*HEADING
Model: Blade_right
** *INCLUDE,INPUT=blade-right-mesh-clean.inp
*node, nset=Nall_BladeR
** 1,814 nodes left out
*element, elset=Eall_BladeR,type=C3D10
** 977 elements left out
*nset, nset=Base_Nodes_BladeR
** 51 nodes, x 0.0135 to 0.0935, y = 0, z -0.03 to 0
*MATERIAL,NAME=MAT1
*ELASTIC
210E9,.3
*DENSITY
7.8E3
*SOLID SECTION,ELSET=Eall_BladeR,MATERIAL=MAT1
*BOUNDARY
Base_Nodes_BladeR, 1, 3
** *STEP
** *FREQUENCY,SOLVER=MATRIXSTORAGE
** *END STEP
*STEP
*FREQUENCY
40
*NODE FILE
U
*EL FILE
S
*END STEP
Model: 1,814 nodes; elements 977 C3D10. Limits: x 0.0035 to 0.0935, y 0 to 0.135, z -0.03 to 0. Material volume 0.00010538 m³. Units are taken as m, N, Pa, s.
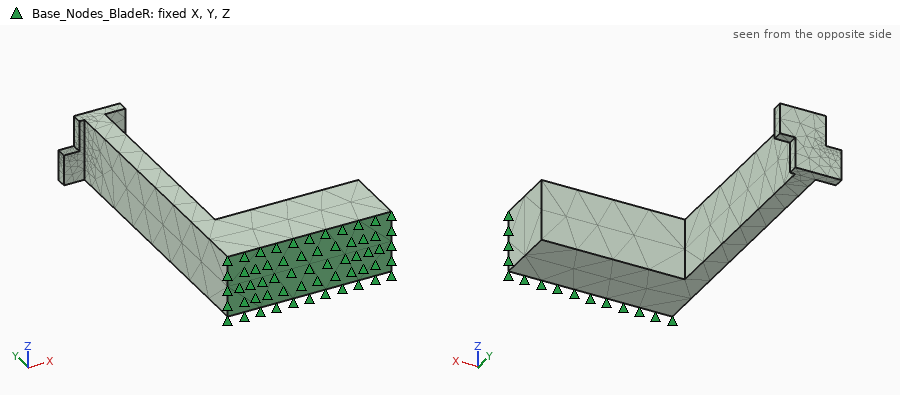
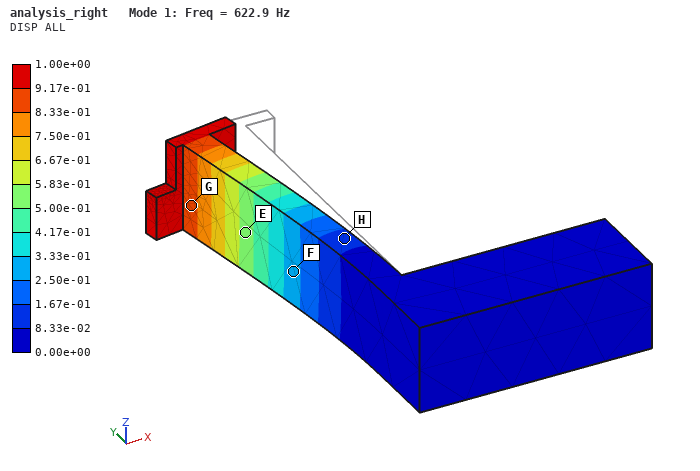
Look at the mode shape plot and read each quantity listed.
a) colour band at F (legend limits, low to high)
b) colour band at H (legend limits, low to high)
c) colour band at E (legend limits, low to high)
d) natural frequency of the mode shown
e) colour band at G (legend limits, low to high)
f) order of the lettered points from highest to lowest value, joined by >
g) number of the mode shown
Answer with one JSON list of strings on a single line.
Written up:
["2.50e-01 to 3.33e-01", "8.33e-02 to 1.67e-01", "5.00e-01 to 5.83e-01", "622.9 Hz", "8.33e-01 to 9.17e-01", "G > E > F > H", "1"]
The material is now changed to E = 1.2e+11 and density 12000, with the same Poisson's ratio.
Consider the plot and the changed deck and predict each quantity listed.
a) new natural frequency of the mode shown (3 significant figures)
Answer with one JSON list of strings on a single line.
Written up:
["380 Hz"]
